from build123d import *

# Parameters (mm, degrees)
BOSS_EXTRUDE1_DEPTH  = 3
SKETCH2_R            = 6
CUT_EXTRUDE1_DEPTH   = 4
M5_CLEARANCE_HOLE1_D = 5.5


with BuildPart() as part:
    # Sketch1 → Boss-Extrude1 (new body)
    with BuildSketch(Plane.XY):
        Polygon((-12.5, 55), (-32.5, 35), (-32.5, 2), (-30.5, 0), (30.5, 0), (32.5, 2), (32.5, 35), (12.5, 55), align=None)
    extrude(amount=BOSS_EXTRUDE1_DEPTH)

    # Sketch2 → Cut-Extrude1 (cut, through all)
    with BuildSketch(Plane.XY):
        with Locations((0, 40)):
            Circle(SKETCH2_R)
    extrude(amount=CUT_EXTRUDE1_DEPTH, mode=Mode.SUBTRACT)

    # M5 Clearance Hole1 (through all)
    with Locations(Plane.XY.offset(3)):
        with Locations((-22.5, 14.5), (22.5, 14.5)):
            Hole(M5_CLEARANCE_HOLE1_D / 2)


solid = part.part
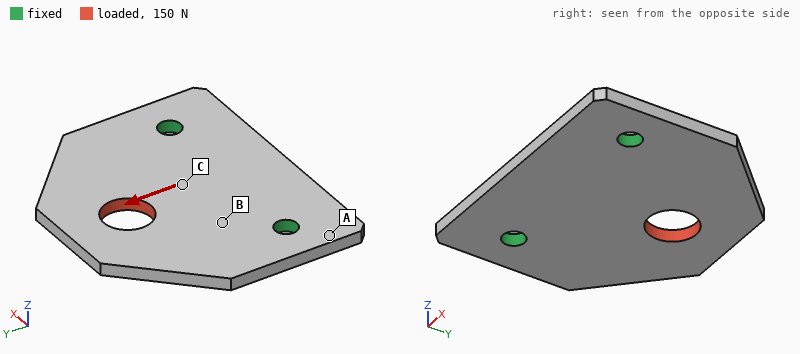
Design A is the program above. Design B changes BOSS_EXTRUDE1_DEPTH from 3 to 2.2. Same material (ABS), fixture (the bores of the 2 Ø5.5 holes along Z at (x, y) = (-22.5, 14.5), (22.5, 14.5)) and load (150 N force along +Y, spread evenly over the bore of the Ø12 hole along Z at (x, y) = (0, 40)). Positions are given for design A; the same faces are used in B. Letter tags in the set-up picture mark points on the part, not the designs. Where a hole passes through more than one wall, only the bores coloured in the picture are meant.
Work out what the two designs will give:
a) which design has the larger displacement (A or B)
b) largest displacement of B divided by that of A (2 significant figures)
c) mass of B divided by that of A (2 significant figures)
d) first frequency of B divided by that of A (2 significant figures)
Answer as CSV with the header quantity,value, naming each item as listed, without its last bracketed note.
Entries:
quantity,value
which design has the larger displacement,B
largest displacement of B divided by that of A,1.4
mass of B divided by that of A,0.73
first frequency of B divided by that of A,0.75
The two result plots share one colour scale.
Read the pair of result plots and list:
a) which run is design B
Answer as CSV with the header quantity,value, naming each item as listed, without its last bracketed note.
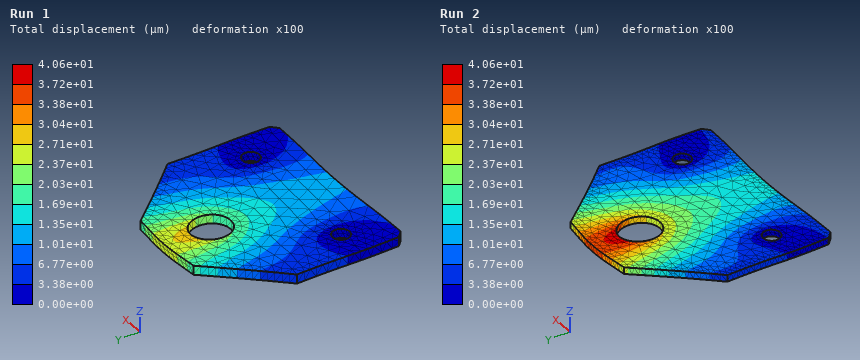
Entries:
quantity,value
which run is design B,Run 2
